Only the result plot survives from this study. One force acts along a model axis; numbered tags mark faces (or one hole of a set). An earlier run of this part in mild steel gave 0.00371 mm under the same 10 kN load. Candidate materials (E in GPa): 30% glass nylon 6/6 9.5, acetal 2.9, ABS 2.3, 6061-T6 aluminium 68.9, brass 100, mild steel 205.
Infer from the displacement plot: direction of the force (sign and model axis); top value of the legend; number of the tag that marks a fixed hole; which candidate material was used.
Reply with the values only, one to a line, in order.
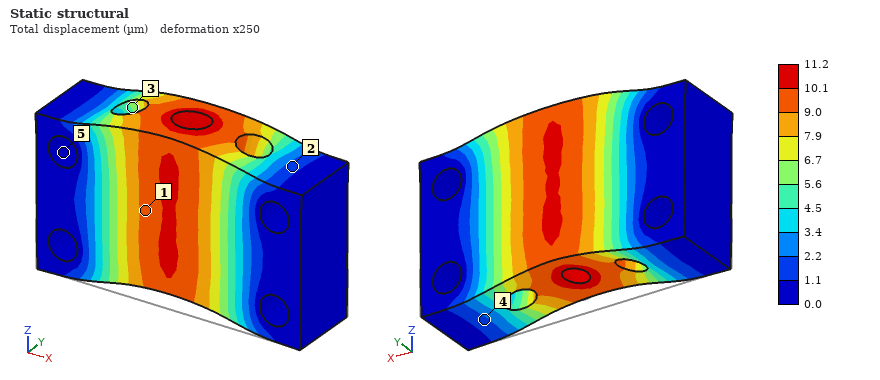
+Z
11.2 µm
5
6061-T6 aluminium
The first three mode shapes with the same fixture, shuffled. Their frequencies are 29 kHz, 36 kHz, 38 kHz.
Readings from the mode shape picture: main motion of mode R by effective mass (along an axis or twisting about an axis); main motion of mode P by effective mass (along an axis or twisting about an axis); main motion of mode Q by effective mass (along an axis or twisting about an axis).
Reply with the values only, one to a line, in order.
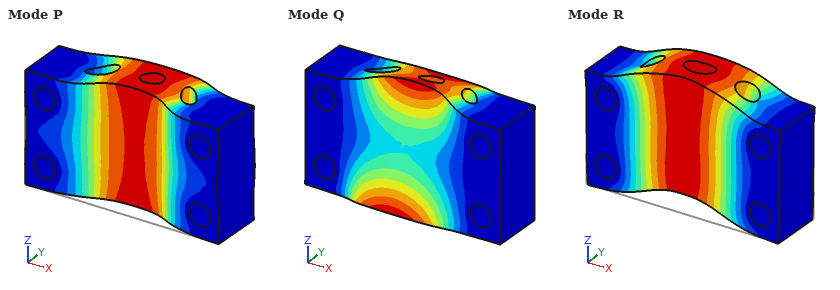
along Z
along Y
twisting about X
